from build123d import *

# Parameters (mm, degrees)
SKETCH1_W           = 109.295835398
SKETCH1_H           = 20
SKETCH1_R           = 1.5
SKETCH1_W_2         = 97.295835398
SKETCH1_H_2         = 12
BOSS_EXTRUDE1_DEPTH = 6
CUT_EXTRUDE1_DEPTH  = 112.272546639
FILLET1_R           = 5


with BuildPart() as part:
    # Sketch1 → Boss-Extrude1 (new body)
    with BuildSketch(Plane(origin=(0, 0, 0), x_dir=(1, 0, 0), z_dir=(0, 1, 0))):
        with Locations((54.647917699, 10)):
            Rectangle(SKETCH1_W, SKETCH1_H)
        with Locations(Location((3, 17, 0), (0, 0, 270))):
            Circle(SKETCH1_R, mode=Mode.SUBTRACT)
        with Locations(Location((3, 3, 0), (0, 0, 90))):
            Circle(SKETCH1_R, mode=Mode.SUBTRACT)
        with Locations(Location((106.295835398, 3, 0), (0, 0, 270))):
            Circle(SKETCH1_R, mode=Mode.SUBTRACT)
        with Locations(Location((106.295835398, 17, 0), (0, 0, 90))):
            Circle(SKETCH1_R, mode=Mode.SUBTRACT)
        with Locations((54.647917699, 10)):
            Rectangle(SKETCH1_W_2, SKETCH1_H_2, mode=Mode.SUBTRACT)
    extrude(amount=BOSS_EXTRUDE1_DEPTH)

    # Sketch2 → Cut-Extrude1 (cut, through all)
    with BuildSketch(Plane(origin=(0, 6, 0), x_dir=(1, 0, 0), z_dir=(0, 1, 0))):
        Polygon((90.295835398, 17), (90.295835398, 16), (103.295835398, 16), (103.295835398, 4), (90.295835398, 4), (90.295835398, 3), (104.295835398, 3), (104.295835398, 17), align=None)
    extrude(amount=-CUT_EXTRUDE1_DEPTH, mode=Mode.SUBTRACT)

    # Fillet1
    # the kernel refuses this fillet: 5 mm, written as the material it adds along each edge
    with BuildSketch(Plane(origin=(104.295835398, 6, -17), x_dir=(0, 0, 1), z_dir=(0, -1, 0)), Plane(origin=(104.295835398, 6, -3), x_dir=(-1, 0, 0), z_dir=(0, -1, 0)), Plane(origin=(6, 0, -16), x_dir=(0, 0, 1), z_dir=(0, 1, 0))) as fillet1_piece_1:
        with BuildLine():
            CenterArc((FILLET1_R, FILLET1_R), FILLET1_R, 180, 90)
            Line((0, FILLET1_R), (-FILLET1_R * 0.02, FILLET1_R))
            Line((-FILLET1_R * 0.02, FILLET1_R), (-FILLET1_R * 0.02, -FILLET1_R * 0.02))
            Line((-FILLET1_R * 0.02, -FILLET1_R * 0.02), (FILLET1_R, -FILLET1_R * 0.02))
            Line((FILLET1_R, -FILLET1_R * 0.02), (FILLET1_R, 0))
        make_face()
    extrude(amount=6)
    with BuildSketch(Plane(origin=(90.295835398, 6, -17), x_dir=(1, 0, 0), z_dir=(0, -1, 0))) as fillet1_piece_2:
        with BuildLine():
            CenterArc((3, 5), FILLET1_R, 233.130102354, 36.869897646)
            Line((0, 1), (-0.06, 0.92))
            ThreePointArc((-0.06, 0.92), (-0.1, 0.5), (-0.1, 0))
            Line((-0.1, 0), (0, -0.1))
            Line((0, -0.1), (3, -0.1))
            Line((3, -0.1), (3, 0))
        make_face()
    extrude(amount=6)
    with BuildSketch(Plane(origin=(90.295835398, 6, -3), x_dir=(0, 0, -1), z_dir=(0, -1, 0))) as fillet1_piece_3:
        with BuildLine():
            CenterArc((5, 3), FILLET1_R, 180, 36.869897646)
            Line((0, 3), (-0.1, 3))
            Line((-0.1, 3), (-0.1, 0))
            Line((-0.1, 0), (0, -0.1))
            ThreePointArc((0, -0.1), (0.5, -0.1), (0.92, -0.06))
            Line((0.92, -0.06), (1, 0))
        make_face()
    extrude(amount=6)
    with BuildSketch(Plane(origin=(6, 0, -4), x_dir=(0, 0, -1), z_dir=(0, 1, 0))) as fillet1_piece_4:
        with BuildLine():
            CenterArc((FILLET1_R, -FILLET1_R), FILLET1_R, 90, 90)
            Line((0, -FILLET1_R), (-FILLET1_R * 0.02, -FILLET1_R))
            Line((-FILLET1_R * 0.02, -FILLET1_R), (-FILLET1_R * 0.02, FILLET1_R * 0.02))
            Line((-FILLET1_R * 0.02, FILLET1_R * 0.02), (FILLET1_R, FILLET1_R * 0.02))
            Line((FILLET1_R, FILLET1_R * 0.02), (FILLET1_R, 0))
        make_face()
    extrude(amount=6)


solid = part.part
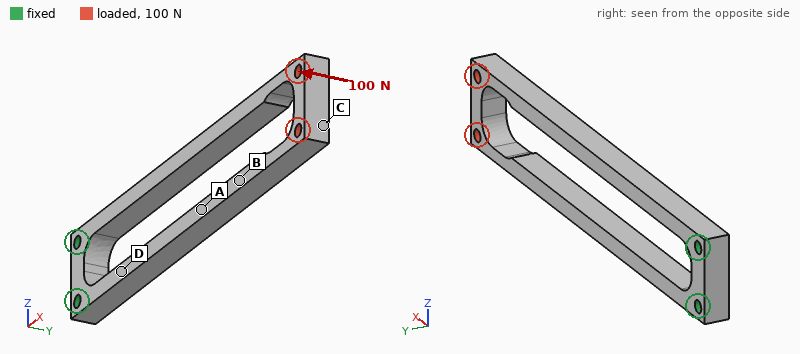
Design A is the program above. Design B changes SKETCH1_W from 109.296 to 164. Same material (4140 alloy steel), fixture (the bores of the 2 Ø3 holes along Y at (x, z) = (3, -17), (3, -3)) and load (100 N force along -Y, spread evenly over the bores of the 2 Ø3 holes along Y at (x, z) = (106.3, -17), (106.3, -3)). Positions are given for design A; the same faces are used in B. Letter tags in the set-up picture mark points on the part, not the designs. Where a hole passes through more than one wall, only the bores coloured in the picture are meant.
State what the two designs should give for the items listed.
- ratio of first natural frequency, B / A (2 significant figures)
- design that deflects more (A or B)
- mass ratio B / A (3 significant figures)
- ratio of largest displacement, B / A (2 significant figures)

0.48
B
2.12
1.4
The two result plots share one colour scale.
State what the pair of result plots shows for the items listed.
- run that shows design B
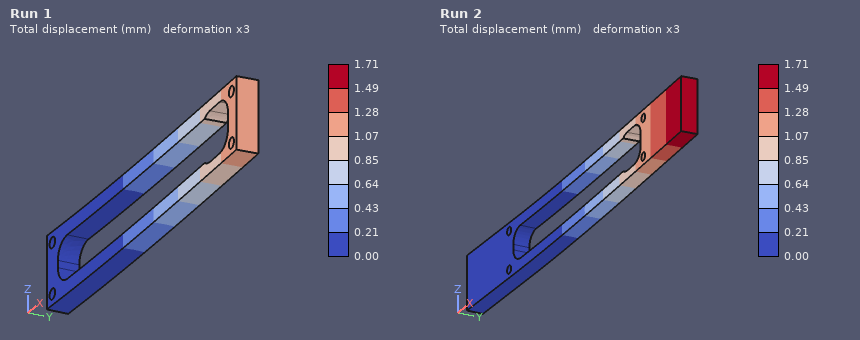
Run 2
